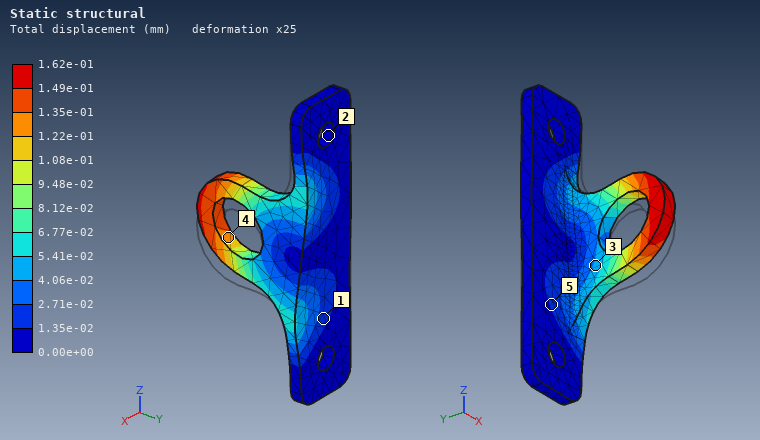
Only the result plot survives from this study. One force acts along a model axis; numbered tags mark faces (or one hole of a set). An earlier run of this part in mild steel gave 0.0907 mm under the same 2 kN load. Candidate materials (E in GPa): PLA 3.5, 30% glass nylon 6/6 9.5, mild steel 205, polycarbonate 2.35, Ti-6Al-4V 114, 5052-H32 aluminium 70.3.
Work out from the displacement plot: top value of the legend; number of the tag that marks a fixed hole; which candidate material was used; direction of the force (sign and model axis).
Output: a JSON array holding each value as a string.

["1.62e-01 mm", "2", "Ti-6Al-4V", "+Z"]
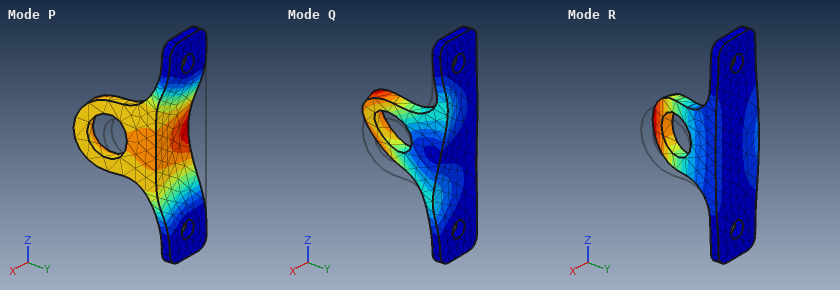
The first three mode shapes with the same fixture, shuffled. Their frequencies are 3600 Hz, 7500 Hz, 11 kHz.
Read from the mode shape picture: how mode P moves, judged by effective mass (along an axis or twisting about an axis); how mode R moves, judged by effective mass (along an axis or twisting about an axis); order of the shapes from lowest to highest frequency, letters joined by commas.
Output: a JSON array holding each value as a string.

["along Y", "along X", "R, P, Q"]
